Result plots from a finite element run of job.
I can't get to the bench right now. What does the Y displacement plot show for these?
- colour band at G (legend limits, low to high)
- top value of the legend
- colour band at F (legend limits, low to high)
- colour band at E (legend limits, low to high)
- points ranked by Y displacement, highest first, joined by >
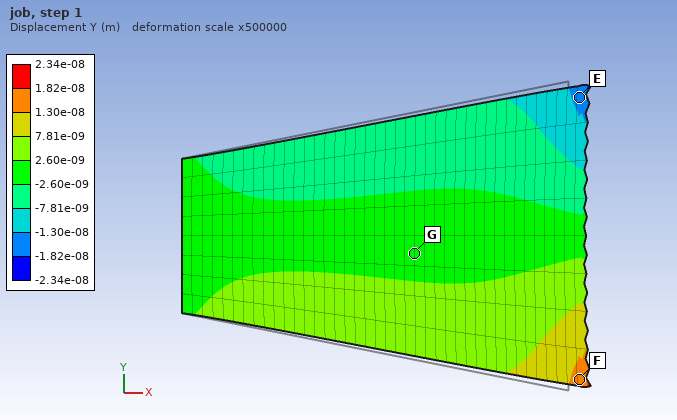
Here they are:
-2.60e-09 to 2.60e-09 m
2.34e-08 m
1.30e-08 to 1.82e-08 m
-1.82e-08 to -1.30e-08 m
F > G > E
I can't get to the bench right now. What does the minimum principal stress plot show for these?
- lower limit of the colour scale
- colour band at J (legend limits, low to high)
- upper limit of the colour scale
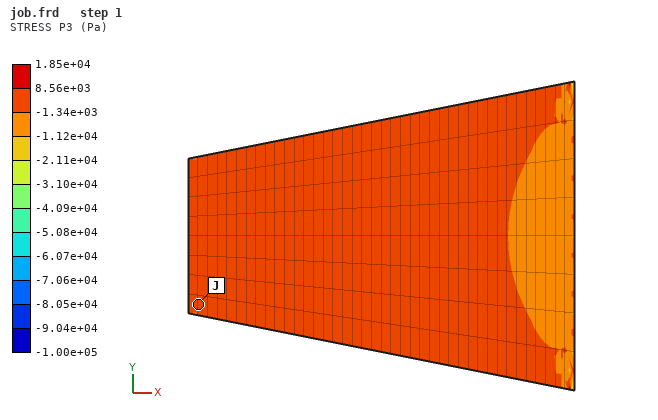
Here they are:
-1.00e+05 Pa
-1.34e+03 to 8.56e+03 Pa
1.85e+04 Pa
